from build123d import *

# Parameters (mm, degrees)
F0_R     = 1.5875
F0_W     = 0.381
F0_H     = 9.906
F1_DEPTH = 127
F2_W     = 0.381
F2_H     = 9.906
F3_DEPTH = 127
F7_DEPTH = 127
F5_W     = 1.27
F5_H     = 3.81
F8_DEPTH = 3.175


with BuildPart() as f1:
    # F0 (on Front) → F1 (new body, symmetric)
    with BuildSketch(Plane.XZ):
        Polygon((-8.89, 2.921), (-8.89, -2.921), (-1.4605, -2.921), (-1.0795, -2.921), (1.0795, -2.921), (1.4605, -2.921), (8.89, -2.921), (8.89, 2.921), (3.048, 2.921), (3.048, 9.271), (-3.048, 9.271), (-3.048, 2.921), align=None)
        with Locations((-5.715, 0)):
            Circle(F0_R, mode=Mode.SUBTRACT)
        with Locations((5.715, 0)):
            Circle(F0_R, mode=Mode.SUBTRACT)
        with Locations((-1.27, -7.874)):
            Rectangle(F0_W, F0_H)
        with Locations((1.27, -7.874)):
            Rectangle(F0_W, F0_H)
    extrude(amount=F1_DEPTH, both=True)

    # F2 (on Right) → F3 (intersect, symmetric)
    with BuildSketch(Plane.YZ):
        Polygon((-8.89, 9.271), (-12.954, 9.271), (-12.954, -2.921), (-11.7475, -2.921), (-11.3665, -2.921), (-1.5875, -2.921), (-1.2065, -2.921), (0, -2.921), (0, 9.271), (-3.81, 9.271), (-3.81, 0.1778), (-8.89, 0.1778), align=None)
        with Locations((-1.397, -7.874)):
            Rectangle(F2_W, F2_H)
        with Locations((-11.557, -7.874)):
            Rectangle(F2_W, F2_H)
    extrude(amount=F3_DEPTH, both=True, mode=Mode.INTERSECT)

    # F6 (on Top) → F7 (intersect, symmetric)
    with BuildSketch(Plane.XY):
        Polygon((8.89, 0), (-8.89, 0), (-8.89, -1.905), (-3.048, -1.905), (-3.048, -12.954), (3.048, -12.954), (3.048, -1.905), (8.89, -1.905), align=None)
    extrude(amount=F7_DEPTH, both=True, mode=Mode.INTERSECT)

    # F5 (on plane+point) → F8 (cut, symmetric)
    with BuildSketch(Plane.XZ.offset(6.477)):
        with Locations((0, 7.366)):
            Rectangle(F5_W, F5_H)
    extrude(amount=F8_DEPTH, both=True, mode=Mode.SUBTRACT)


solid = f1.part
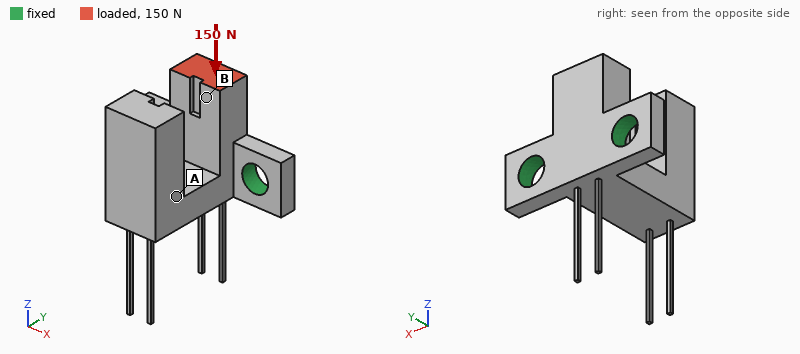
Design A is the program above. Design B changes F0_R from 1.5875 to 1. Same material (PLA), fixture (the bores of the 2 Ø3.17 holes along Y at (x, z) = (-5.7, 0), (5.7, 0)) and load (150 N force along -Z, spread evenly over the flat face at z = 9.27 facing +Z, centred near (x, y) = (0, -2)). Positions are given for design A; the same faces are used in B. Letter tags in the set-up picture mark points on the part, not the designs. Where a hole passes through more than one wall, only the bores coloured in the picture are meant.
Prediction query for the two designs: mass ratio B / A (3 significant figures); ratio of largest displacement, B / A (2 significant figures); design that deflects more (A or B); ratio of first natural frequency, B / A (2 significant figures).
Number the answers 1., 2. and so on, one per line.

1. 1.02
2. 1.5
3. B
4. 1.0
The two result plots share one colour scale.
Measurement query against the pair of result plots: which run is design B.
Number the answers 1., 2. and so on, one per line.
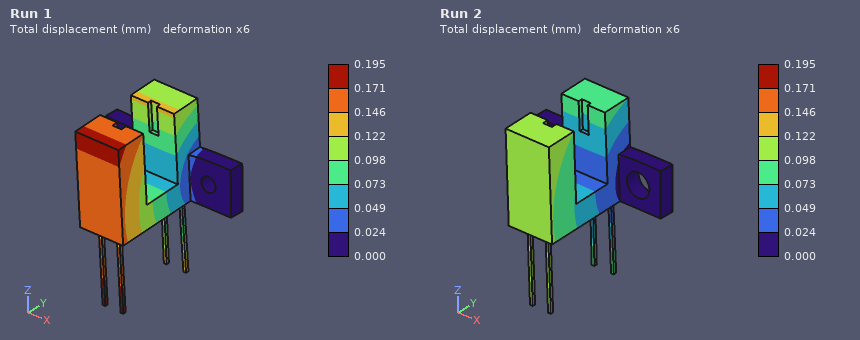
1. Run 1
